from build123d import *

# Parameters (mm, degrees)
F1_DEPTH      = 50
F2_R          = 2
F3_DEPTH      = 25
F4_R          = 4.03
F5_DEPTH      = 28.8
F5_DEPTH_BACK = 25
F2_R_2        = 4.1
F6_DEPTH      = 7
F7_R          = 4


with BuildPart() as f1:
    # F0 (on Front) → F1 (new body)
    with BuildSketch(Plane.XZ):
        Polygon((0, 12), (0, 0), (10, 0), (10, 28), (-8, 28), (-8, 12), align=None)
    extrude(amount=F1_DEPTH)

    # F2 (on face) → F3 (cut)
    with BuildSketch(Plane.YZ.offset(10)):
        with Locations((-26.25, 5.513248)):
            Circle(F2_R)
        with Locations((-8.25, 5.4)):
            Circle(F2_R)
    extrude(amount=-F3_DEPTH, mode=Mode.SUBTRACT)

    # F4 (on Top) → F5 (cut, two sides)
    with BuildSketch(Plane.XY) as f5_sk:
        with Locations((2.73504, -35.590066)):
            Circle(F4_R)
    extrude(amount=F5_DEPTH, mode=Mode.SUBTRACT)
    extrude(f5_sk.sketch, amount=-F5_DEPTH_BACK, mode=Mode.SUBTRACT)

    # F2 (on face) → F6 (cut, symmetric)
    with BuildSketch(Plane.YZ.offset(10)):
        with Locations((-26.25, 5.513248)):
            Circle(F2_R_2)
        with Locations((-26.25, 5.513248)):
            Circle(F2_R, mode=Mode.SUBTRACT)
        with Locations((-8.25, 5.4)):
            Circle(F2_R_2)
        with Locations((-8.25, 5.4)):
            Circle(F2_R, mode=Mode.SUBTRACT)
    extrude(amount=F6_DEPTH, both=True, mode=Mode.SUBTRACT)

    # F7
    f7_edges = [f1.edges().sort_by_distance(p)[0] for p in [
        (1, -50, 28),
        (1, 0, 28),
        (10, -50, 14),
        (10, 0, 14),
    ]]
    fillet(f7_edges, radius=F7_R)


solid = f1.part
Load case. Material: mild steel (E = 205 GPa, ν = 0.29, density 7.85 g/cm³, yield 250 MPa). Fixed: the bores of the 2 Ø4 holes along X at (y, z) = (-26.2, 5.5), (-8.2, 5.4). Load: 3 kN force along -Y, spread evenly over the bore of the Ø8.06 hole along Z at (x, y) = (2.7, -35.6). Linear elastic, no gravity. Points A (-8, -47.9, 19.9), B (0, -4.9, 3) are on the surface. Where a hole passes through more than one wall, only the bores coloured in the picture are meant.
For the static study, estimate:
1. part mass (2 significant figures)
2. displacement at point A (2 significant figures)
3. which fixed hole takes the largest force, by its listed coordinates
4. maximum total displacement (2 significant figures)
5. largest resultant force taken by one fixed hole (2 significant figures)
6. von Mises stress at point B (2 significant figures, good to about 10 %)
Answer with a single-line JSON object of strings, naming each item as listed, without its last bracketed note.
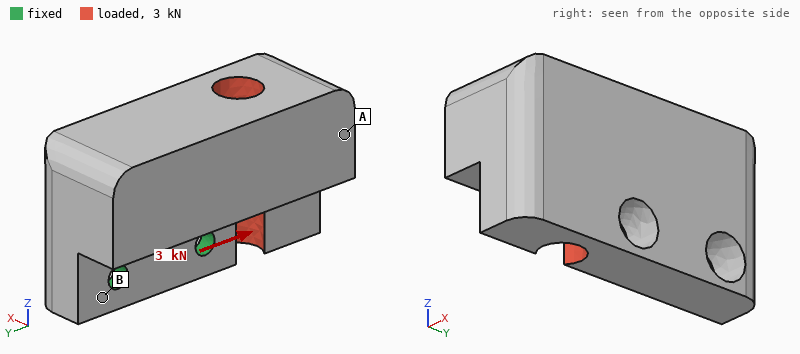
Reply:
{"part mass": "140 g", "displacement at point A": "5.8 µm", "which fixed hole takes the largest force, by its listed coordinates": "(-26.2, 5.5)", "maximum total displacement": "7.0 µm", "largest resultant force taken by one fixed hole": "2.2 kN", "von Mises stress at point B": "27 MPa"}
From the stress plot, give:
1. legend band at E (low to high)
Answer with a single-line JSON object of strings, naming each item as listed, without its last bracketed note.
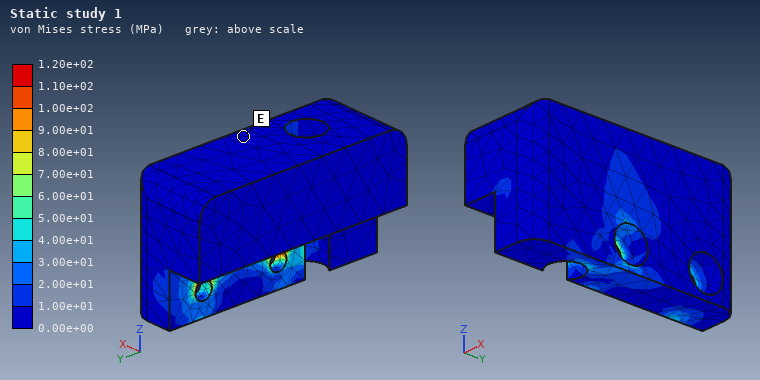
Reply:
{"legend band at E": "0.00e+00 to 1.00e+01 MPa"}
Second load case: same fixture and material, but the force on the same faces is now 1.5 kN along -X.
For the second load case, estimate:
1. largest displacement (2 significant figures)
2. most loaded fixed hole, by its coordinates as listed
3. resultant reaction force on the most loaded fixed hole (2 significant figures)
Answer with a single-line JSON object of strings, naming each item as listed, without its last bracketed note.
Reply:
{"largest displacement": "41 µm", "most loaded fixed hole, by its coordinates as listed": "(-26.2, 5.5)", "resultant reaction force on the most loaded fixed hole": "2.1 kN"}
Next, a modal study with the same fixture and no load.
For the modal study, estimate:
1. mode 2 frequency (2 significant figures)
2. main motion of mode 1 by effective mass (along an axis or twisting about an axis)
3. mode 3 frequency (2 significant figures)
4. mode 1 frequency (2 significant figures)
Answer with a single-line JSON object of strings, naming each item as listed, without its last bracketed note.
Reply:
{"mode 2 frequency": "6600 Hz", "main motion of mode 1 by effective mass": "along X", "mode 3 frequency": "8000 Hz", "mode 1 frequency": "3200 Hz"}
